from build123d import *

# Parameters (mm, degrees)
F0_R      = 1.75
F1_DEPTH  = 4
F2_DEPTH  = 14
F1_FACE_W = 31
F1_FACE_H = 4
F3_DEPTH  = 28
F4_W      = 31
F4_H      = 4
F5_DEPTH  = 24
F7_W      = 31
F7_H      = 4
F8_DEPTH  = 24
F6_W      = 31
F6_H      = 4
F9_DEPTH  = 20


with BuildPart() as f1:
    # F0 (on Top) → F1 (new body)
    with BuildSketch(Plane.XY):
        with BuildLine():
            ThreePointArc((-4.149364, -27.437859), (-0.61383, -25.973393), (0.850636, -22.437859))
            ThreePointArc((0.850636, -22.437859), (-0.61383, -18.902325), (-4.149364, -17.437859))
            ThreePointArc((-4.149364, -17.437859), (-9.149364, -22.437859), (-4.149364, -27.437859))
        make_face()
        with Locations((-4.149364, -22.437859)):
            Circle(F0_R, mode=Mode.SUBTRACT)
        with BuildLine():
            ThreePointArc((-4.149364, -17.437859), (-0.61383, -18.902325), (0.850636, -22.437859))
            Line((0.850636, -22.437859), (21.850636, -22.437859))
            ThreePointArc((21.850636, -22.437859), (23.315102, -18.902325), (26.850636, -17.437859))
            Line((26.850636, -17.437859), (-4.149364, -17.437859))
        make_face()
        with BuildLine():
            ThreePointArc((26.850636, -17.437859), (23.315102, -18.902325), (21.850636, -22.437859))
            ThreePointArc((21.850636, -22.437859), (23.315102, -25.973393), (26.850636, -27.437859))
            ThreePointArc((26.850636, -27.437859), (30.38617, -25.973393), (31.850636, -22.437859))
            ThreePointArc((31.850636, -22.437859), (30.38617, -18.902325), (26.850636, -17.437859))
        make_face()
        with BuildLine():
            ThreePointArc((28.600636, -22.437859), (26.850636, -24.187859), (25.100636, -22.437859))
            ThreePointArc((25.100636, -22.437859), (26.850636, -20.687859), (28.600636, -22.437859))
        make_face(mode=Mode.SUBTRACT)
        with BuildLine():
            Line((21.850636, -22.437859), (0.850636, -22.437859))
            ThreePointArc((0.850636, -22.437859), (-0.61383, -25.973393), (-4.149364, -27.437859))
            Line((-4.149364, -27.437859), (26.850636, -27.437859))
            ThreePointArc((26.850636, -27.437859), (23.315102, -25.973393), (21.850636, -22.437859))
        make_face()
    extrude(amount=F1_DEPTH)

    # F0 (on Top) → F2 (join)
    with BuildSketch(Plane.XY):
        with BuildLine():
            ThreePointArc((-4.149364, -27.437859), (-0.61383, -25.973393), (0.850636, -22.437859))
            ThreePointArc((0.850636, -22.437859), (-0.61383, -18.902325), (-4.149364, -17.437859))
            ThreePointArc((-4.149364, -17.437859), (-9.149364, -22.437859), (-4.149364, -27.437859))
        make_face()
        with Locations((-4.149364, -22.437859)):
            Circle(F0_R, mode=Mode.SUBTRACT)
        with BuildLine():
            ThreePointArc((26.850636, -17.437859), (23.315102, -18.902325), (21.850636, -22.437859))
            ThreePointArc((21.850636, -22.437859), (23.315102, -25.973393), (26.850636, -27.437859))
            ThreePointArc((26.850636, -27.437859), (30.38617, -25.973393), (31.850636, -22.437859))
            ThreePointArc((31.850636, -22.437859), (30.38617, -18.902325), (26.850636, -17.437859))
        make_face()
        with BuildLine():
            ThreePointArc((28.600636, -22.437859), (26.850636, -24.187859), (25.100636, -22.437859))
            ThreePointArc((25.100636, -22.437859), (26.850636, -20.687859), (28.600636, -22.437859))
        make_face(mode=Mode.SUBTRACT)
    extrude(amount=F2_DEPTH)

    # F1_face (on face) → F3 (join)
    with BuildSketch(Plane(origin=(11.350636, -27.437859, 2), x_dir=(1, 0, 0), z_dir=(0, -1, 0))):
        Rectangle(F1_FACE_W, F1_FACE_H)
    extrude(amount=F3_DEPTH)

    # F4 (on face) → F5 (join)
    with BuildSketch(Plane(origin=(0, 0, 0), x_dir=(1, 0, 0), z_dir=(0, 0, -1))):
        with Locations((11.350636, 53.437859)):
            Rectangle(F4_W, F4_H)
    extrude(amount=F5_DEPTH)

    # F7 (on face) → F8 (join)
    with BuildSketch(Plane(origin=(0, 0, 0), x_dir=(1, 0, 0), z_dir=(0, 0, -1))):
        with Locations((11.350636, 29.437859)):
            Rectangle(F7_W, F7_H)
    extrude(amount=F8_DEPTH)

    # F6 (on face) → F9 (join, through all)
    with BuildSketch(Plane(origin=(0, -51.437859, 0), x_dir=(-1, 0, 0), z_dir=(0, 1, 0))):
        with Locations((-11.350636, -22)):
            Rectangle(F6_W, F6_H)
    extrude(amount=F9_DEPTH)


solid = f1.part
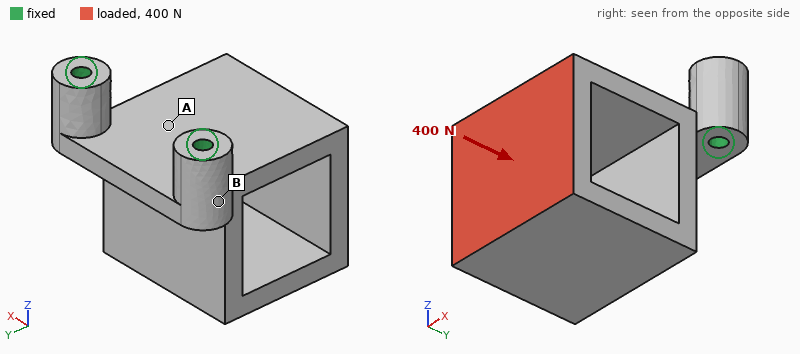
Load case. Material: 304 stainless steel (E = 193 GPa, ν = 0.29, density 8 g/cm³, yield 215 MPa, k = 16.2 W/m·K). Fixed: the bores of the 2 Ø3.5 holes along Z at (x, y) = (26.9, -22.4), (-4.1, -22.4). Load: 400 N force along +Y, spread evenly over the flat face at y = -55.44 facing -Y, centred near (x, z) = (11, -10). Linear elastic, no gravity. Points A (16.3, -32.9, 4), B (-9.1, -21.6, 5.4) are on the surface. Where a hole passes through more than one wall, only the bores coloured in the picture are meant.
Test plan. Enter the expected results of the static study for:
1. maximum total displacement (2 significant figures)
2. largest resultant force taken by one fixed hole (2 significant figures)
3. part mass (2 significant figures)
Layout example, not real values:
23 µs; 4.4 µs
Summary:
51 µm; 220 N; 120 g
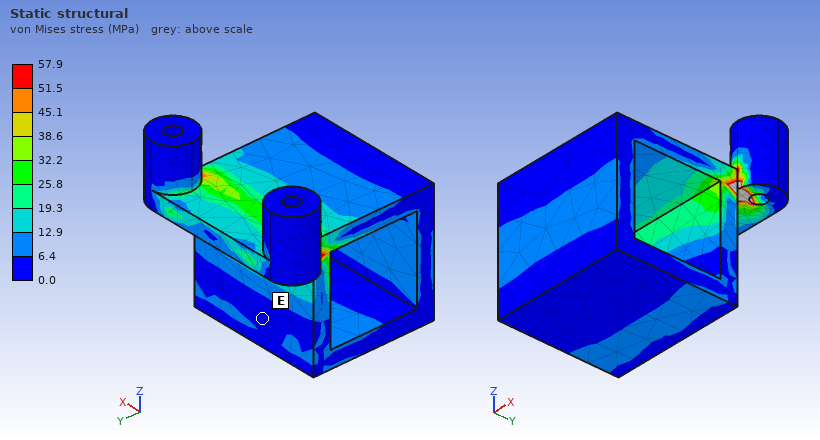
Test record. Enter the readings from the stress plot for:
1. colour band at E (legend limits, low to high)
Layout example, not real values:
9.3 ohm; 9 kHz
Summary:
0.0 to 6.4 MPa
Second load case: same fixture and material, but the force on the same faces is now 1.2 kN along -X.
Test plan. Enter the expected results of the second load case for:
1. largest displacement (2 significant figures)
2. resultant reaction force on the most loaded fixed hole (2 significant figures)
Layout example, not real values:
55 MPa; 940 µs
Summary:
39 µm; 1.5 kN
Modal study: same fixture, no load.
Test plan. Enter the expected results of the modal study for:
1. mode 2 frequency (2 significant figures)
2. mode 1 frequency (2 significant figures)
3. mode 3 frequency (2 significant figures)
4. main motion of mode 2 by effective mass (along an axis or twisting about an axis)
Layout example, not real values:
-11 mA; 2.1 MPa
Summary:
4700 Hz; 1300 Hz; 6100 Hz; along X
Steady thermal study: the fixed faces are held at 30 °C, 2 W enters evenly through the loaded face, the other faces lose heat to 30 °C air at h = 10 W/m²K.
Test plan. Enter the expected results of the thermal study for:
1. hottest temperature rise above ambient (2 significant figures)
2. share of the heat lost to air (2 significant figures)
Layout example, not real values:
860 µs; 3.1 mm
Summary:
20 K; 37 %
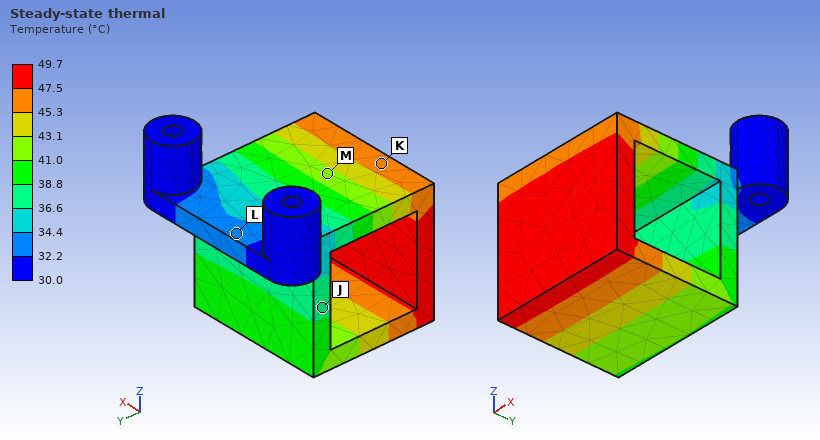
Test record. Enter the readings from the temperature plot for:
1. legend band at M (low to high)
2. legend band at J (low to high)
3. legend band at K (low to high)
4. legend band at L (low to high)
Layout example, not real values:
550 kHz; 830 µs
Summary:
41.0 to 43.1 °C; 36.6 to 38.8 °C; 45.3 to 47.5 °C; 32.2 to 34.4 °C
